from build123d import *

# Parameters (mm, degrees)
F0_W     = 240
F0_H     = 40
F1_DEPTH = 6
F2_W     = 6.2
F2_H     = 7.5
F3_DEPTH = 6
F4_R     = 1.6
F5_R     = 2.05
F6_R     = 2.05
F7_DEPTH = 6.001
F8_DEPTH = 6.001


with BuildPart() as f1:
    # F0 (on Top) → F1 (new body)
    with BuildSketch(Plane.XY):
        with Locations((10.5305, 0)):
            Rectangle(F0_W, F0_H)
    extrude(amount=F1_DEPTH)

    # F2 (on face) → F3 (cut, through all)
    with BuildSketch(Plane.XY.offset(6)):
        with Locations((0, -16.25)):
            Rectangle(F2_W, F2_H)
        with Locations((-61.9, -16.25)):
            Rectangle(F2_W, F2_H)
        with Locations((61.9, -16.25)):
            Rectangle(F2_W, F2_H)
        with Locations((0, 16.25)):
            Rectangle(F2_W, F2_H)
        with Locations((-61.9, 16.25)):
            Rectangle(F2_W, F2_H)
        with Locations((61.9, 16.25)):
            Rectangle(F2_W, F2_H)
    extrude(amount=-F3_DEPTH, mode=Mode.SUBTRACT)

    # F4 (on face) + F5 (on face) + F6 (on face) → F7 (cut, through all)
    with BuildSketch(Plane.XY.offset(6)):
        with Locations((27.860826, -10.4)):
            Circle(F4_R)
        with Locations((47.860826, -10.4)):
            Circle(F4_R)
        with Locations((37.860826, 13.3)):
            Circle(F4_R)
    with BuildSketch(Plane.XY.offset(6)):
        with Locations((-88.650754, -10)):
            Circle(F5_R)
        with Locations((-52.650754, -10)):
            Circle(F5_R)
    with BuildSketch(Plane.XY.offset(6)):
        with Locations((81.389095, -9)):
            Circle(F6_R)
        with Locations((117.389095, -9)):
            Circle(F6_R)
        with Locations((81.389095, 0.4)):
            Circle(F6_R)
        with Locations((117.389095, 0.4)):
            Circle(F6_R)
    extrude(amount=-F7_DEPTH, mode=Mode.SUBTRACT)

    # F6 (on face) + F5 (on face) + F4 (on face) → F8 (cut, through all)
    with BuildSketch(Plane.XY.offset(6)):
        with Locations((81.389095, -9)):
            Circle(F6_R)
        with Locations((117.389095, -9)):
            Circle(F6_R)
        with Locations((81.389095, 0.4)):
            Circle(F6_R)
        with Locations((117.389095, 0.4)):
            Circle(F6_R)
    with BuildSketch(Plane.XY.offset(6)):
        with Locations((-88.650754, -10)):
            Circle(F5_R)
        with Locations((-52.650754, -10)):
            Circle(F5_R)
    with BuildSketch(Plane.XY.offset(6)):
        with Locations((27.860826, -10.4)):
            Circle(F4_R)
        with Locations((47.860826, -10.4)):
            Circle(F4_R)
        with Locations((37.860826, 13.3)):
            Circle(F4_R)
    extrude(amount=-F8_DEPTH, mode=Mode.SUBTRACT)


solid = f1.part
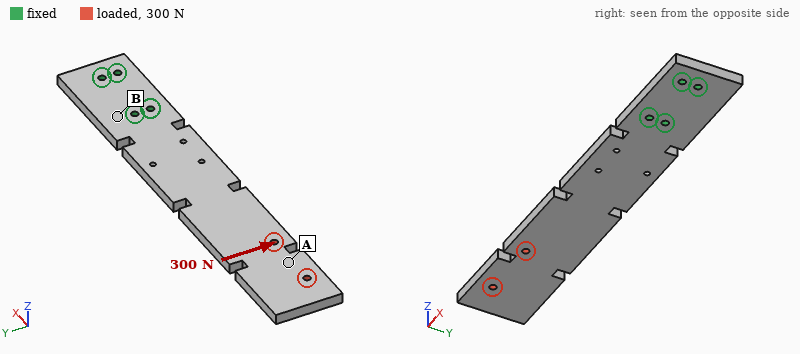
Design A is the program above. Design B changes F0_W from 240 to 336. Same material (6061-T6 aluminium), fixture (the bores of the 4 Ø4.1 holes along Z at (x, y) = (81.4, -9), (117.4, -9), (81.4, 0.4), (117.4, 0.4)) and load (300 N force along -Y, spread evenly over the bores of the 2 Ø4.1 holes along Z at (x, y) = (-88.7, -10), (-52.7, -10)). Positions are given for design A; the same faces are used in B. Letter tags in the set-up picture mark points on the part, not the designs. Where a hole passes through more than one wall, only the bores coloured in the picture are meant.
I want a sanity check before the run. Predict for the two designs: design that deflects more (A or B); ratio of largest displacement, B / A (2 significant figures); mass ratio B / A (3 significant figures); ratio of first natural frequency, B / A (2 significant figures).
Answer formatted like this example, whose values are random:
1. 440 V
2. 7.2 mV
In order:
1. B
2. 1.3
3. 1.42
4. 0.63
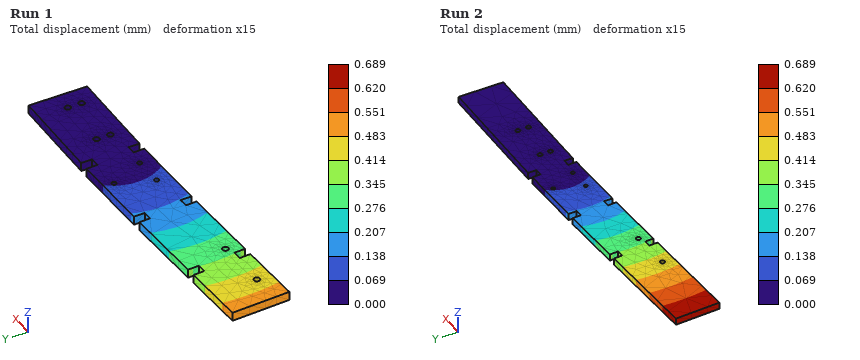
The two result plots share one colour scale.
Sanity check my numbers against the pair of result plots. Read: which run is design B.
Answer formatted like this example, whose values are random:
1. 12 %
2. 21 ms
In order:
1. Run 2
